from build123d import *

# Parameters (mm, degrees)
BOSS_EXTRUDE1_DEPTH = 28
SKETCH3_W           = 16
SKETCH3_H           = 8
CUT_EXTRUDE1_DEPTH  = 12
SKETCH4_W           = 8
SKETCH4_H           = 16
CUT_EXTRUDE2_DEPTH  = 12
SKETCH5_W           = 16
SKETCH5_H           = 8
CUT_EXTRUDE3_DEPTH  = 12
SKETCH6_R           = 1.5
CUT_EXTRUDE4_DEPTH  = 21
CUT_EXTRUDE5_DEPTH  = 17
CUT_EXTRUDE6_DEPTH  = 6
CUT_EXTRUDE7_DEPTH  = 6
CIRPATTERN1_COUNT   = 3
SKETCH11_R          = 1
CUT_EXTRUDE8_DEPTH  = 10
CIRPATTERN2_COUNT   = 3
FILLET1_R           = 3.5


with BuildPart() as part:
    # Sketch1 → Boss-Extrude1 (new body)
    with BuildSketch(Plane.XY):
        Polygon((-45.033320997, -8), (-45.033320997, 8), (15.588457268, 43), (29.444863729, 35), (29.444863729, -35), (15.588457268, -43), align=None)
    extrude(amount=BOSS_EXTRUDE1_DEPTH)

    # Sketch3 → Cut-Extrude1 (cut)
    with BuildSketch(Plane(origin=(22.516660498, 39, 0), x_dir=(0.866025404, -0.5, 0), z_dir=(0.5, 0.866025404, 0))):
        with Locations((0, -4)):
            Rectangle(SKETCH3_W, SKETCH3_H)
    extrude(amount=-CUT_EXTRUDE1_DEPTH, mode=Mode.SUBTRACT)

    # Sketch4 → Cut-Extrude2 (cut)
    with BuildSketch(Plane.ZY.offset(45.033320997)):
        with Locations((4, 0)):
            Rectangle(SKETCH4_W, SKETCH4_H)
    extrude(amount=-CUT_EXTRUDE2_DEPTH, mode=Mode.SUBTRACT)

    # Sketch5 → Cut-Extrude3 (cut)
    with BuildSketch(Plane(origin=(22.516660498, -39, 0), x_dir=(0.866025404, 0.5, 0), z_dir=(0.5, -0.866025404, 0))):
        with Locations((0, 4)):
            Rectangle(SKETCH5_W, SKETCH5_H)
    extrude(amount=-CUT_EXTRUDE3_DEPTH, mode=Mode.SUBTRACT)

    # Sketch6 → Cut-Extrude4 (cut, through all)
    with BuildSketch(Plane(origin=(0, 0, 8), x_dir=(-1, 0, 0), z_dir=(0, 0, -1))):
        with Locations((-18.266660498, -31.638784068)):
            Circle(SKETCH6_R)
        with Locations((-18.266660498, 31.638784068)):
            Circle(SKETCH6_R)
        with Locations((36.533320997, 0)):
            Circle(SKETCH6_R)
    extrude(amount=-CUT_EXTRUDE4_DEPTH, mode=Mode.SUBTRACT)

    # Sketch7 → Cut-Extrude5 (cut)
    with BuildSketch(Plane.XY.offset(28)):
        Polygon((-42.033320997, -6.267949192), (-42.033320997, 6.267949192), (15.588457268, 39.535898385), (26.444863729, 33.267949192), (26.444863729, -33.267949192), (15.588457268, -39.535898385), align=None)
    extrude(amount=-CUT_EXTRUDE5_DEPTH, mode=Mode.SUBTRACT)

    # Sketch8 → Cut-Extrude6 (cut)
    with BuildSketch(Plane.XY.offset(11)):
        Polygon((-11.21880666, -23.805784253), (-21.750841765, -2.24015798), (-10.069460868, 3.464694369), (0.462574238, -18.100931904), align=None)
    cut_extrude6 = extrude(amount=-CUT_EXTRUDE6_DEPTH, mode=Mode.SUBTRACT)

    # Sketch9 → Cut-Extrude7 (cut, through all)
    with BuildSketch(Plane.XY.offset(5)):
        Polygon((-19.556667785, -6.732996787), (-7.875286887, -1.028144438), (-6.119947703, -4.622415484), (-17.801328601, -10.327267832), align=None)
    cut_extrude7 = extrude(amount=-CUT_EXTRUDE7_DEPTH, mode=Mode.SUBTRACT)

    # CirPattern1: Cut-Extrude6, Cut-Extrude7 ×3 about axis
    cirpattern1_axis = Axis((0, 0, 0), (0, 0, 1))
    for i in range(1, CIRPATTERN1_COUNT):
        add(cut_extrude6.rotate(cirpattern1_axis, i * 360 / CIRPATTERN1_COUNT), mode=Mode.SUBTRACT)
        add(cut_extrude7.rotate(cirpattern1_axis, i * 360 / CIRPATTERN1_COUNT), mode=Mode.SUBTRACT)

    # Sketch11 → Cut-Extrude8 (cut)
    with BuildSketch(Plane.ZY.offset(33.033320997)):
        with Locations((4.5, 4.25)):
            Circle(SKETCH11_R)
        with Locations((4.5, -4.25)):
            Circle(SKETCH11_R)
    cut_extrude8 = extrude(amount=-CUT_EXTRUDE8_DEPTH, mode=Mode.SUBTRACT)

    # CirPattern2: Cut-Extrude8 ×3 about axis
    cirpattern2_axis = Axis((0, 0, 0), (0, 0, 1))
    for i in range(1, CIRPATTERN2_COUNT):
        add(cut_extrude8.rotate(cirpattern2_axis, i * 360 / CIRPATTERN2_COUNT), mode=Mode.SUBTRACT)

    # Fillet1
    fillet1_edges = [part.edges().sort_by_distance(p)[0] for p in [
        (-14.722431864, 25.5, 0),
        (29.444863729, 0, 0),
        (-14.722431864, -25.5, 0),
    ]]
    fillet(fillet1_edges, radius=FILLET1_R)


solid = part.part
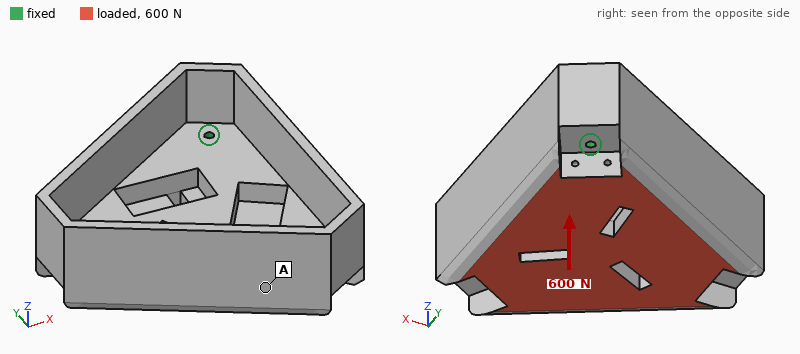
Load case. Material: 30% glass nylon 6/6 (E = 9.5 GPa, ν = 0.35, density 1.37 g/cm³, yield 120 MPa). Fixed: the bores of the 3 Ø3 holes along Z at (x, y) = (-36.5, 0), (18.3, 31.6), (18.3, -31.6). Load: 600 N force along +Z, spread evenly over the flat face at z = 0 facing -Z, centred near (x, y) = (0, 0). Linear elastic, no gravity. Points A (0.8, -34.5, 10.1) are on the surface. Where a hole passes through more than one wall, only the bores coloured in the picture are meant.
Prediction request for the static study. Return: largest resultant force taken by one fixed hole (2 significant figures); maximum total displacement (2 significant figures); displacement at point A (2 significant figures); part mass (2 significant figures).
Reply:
230 N
29 µm
13 µm
64 g
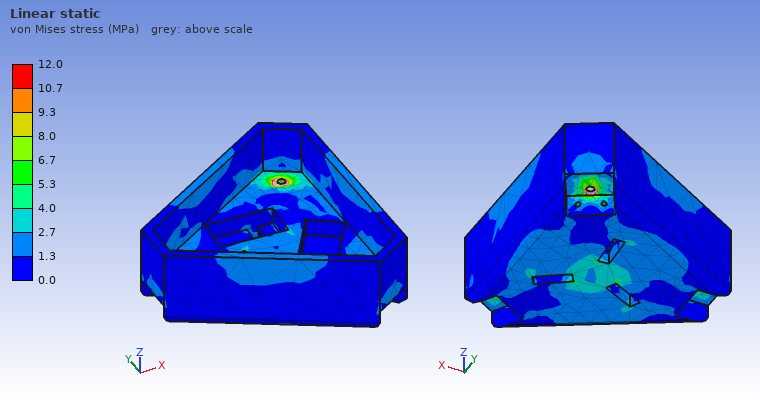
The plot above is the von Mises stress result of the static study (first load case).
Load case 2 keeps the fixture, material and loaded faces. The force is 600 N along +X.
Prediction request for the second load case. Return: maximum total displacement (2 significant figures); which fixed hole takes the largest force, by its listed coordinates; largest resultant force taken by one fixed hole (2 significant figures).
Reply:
14 µm
(-36.5, 0)
260 N
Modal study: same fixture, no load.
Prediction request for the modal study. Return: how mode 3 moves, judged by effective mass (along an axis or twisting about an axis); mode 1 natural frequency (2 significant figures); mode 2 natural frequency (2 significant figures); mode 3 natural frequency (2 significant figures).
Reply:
along Z
3000 Hz
3000 Hz
3900 Hz
